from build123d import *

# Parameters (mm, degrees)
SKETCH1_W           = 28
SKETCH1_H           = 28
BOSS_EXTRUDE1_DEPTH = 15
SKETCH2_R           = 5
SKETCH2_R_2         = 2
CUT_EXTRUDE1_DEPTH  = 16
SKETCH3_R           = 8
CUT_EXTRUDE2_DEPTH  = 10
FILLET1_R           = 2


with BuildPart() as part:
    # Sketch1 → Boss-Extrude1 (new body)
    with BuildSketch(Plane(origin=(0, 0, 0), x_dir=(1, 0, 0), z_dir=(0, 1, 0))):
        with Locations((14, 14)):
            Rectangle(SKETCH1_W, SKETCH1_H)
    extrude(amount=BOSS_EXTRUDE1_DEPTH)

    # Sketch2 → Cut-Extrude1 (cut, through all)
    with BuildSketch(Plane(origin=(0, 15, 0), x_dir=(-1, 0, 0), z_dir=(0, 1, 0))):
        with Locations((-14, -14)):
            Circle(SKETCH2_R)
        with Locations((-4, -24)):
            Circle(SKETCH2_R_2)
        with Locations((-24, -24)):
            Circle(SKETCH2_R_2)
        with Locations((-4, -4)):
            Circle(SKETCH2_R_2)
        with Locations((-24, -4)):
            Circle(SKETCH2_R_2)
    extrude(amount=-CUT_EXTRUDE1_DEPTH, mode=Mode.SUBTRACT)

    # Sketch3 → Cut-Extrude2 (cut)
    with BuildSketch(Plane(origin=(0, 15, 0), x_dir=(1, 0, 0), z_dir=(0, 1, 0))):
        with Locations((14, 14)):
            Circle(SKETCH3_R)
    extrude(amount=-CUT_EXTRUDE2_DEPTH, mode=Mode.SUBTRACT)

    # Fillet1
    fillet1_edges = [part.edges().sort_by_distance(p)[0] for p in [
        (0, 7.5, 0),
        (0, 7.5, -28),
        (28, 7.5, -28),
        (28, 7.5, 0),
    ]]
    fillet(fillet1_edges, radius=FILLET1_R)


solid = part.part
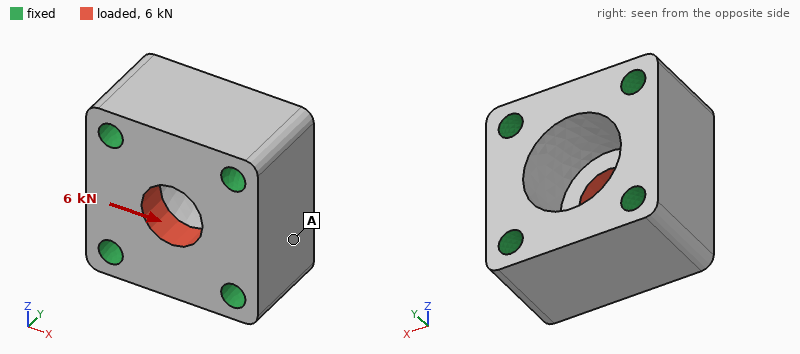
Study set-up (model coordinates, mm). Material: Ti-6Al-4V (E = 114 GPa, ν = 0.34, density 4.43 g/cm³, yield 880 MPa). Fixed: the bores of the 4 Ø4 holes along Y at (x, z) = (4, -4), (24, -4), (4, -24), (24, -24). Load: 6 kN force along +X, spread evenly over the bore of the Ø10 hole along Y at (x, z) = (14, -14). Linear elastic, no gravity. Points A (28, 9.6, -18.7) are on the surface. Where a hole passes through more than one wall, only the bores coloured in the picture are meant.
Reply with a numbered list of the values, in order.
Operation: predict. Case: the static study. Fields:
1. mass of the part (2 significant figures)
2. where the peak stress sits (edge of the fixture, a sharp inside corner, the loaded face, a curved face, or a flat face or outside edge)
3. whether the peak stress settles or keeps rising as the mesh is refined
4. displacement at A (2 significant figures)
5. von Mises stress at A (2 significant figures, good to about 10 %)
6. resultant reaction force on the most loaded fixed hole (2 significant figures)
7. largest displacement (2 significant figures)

1. 38 g
2. edge of the fixture
3. keeps rising
4. 0.71 µm
5. 9.6 MPa
6. 1.6 kN
7. 4.7 µm
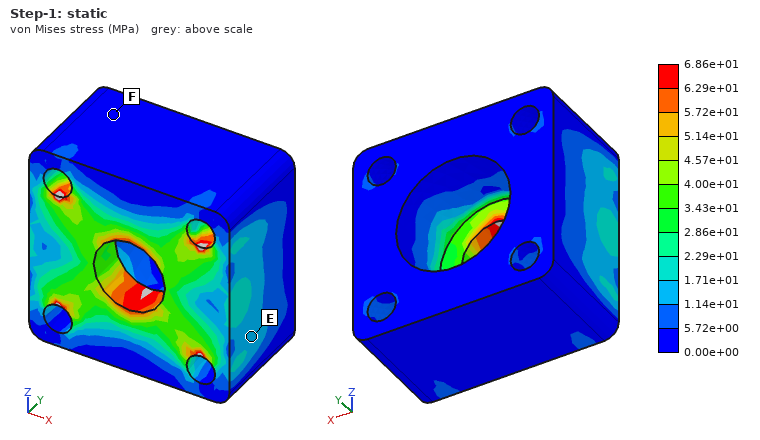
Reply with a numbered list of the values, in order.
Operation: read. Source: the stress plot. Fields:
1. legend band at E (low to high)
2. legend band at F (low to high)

1. 1.14e+01 to 1.71e+01 MPa
2. 0.00e+00 to 5.72e+00 MPa
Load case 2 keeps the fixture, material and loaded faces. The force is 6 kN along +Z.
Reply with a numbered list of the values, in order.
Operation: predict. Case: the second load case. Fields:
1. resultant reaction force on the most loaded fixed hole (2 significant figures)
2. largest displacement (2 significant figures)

1. 1.6 kN
2. 4.6 µm
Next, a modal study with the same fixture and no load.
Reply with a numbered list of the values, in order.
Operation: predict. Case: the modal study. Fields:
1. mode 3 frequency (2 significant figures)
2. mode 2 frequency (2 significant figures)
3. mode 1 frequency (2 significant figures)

1. 76 kHz
2. 75 kHz
3. 61 kHz
